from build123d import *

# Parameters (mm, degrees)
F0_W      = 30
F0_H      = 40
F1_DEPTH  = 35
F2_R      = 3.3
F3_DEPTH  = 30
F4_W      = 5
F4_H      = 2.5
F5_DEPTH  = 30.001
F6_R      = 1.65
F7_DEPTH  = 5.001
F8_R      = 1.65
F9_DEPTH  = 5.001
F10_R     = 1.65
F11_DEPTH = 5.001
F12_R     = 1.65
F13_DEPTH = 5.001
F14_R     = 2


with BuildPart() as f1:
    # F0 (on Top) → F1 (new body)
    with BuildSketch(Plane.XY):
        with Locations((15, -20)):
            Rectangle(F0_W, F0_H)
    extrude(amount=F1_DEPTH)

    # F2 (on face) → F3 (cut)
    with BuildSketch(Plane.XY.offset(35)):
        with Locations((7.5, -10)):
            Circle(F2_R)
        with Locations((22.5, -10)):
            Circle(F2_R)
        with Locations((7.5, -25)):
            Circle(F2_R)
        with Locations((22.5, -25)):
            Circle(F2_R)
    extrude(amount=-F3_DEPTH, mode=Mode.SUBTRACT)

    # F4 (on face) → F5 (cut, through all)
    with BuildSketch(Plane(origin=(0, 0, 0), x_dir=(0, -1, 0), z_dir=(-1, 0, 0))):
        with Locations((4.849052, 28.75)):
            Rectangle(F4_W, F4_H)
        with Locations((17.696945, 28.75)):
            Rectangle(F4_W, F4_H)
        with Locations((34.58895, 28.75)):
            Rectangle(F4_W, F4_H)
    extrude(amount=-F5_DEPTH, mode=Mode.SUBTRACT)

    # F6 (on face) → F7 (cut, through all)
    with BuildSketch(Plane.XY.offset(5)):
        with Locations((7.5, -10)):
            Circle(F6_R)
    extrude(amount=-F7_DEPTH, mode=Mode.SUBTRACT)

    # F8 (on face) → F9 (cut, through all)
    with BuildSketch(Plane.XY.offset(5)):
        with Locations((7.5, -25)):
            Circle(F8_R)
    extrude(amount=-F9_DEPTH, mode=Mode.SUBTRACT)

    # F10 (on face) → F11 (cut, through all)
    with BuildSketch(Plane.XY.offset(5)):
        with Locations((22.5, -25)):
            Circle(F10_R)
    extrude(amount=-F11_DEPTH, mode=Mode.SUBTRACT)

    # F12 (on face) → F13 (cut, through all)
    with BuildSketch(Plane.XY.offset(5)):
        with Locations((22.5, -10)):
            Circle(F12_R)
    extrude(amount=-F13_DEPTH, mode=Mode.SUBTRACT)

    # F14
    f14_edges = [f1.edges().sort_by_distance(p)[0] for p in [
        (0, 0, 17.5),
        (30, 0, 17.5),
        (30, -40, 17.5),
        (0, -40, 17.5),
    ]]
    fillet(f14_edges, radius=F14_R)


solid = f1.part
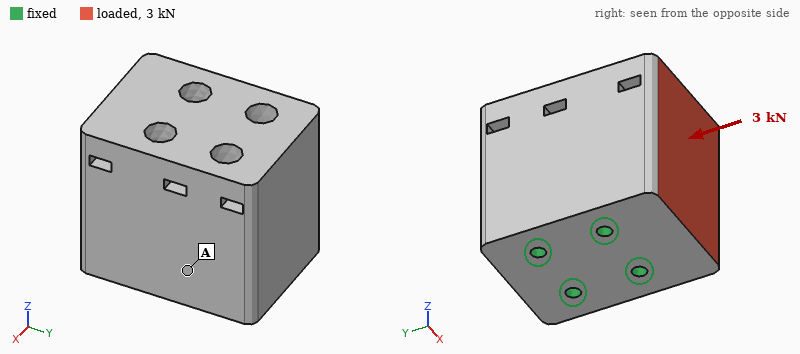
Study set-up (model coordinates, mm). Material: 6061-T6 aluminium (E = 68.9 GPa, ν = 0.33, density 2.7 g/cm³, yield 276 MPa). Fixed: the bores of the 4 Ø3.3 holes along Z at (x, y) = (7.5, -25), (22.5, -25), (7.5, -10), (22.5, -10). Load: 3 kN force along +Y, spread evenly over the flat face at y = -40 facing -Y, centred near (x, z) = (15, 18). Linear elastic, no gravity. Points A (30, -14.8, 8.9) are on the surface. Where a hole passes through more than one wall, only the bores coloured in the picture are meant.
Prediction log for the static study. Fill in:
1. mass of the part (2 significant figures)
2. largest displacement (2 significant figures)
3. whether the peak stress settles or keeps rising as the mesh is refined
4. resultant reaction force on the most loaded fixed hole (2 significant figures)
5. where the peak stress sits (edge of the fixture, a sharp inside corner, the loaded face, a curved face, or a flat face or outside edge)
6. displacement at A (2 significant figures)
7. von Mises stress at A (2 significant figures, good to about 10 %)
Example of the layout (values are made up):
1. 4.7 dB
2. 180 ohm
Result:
1. 99 g
2. 20 µm
3. keeps rising
4. 1.5 kN
5. edge of the fixture
6. 3.5 µm
7. 9.8 MPa
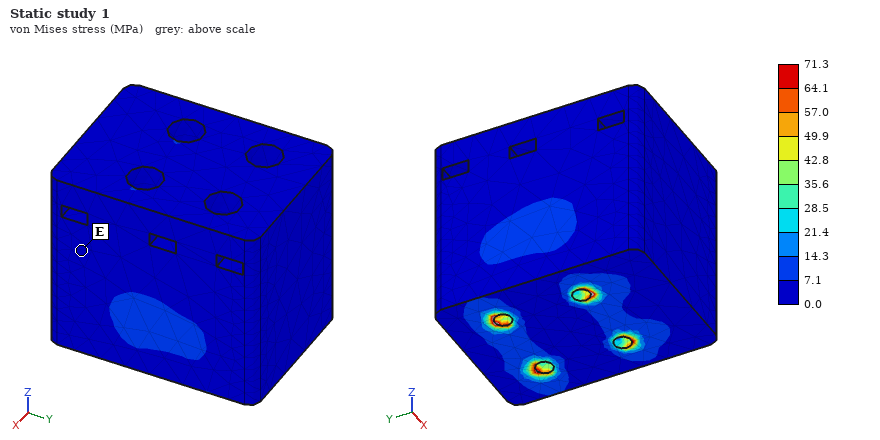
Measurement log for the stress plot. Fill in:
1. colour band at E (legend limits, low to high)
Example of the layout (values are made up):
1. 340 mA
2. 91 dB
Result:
1. 0.0 to 7.1 MPa
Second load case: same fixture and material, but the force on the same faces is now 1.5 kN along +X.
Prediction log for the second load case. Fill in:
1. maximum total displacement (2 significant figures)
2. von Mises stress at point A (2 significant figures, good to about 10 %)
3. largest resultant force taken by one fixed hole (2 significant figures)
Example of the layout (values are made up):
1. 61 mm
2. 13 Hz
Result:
1. 13 µm
2. 7.4 MPa
3. 1.3 kN
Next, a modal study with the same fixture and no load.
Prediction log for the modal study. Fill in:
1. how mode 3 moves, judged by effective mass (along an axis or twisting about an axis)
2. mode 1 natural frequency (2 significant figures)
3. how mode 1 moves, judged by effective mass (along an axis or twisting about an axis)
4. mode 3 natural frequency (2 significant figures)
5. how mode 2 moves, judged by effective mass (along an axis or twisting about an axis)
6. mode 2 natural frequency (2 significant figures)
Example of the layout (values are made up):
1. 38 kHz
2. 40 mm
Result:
1. twisting about Z
2. 7400 Hz
3. along Y
4. 15 kHz
5. along X
6. 8100 Hz
